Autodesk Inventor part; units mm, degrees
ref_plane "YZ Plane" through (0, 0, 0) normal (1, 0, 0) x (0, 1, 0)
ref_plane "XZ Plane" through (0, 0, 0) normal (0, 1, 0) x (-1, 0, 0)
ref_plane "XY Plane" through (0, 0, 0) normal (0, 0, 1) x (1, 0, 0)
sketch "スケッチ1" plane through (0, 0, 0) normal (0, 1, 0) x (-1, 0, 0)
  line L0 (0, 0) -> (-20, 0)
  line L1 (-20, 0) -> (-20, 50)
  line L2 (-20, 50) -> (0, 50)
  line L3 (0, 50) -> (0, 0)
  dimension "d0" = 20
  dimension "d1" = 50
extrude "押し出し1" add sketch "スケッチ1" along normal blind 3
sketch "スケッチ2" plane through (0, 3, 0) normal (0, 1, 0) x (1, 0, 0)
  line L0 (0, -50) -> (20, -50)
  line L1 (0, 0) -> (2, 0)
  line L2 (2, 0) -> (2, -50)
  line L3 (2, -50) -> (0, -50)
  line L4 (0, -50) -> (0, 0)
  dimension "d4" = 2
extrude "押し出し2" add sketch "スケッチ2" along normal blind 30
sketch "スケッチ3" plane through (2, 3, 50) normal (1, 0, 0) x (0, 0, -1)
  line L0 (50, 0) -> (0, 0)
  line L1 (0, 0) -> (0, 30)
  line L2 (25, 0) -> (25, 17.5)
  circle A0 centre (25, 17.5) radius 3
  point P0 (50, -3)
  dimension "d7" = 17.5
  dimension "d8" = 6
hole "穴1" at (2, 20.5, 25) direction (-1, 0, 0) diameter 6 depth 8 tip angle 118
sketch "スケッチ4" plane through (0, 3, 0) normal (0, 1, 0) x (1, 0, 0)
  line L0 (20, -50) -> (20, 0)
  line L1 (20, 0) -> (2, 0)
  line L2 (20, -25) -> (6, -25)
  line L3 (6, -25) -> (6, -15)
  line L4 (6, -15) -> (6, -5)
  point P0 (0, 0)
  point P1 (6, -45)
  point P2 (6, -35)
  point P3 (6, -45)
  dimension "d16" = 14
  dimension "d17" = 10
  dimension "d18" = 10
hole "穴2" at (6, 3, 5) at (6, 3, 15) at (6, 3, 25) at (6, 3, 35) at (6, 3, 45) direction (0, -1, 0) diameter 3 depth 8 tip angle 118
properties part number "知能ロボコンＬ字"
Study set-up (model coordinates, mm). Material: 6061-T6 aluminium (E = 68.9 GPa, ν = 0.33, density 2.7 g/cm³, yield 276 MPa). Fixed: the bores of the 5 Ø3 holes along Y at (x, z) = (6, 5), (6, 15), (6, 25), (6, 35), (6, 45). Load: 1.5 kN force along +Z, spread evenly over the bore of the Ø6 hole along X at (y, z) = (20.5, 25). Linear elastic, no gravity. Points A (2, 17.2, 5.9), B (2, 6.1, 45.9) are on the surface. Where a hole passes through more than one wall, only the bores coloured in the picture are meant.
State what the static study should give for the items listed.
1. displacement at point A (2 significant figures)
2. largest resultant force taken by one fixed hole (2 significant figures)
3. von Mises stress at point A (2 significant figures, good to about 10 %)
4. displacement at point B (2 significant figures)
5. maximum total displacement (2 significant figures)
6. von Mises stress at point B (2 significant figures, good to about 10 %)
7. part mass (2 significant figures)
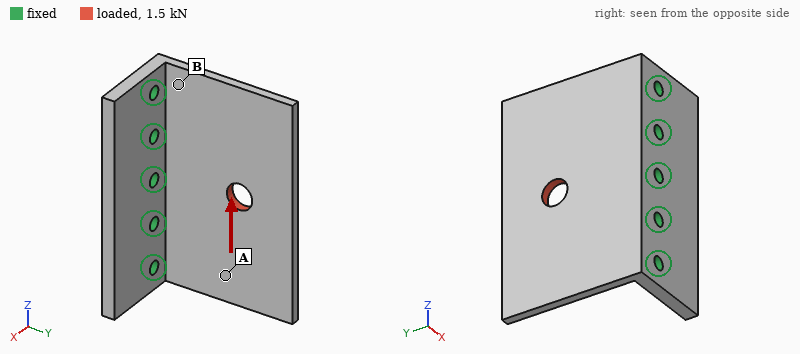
40 µm
640 N
19 MPa
20 µm
70 µm
45 MPa
16 g
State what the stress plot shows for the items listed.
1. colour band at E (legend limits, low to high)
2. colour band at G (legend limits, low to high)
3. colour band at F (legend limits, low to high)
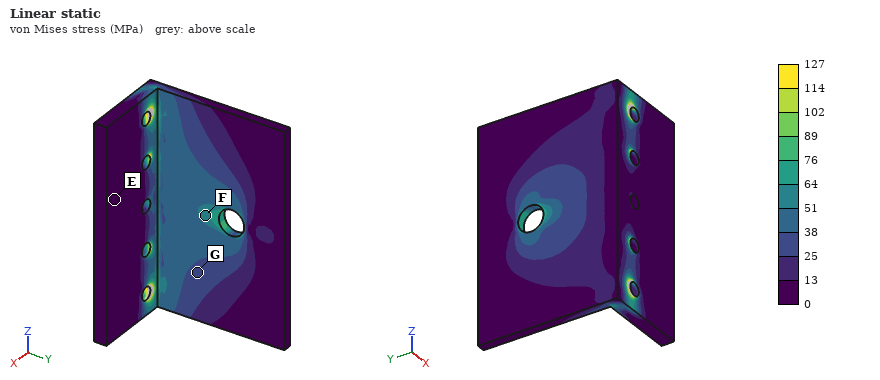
0 to 13 MPa
25 to 38 MPa
51 to 64 MPa
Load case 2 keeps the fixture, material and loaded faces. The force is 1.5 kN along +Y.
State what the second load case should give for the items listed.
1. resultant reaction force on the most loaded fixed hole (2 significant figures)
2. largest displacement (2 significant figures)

360 N
72 µm
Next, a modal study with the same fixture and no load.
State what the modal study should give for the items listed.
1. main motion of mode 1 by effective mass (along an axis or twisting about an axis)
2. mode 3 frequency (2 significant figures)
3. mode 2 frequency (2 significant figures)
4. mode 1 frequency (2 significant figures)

along X
6300 Hz
2800 Hz
1700 Hz
